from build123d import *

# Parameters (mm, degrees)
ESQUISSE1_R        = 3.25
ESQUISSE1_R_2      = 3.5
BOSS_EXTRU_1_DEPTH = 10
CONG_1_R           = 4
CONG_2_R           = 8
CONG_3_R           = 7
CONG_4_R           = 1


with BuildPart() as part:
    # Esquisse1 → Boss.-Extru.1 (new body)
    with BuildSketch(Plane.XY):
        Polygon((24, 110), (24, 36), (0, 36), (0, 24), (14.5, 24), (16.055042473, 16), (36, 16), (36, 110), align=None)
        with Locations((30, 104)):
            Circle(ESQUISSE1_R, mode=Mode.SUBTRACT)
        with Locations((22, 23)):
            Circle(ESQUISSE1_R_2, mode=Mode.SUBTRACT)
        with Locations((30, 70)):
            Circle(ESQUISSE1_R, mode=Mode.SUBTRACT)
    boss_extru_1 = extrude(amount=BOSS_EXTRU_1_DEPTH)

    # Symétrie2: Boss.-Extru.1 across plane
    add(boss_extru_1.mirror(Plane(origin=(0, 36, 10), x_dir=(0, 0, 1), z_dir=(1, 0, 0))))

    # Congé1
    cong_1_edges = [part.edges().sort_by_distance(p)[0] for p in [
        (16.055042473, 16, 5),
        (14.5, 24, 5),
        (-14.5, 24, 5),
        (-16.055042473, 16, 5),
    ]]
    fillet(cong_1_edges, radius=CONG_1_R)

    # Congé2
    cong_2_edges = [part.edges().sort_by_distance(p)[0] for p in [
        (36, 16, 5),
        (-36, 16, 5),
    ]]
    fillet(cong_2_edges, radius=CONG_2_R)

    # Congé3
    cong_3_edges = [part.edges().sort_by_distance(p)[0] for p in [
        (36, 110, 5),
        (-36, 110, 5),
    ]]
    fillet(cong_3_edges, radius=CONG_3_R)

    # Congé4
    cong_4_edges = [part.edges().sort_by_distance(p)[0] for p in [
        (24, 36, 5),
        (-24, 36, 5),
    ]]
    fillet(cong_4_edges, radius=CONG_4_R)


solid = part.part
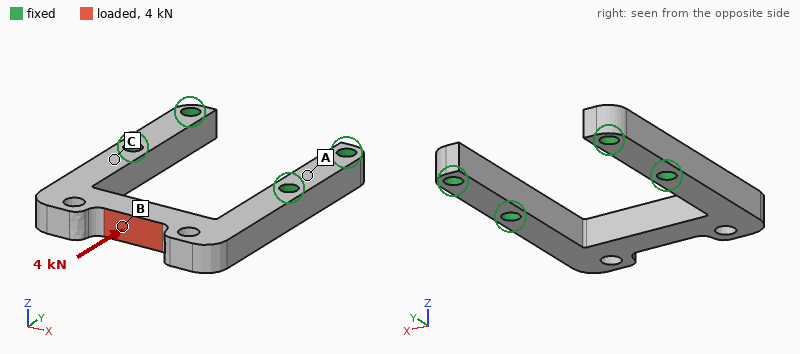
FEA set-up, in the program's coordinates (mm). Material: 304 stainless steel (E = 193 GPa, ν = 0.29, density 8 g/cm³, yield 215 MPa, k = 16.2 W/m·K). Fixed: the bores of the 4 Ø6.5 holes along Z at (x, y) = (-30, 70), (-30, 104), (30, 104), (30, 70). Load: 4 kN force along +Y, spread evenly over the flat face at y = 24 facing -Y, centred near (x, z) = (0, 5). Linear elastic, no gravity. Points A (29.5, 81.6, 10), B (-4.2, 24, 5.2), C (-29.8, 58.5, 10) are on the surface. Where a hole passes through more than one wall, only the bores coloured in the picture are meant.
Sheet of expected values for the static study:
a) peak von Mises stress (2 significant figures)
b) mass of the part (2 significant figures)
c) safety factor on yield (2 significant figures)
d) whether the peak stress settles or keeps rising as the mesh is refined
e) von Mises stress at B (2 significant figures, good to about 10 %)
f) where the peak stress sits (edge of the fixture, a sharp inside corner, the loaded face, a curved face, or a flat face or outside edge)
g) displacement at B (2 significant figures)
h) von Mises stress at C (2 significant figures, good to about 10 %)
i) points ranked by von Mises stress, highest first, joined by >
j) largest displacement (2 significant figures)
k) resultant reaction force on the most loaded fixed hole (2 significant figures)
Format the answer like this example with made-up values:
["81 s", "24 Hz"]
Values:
["250 MPa", "220 g", "0.86", "settles", "100 MPa", "a curved face", "28 µm", "27 MPa", "B > C > A", "30 µm", "2.2 kN"]
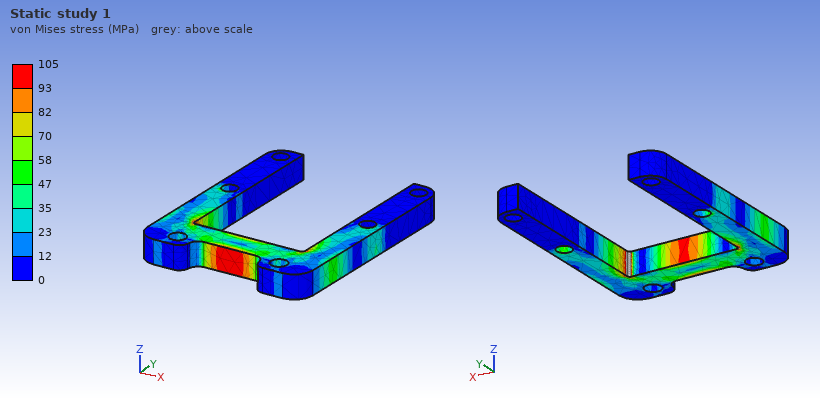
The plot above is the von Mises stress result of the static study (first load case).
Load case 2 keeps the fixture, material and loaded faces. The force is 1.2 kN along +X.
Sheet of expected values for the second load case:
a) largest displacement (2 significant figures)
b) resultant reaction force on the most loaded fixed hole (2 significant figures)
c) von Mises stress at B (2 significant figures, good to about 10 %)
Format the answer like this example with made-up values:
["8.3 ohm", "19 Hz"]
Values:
["19 µm", "800 N", "9.4 MPa"]
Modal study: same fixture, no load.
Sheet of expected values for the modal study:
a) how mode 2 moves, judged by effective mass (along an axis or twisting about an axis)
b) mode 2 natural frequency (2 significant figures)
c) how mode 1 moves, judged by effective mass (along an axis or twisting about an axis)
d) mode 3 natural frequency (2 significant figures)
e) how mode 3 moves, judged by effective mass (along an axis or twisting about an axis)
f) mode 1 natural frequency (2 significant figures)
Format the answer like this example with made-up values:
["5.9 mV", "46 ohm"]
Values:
["twisting about Y", "3800 Hz", "along Z", "4000 Hz", "along X", "2100 Hz"]
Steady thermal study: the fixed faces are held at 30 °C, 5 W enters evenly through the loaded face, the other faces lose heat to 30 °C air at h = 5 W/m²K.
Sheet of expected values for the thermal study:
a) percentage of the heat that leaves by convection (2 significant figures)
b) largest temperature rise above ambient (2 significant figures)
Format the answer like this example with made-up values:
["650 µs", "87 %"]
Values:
["22 %", "65 K"]
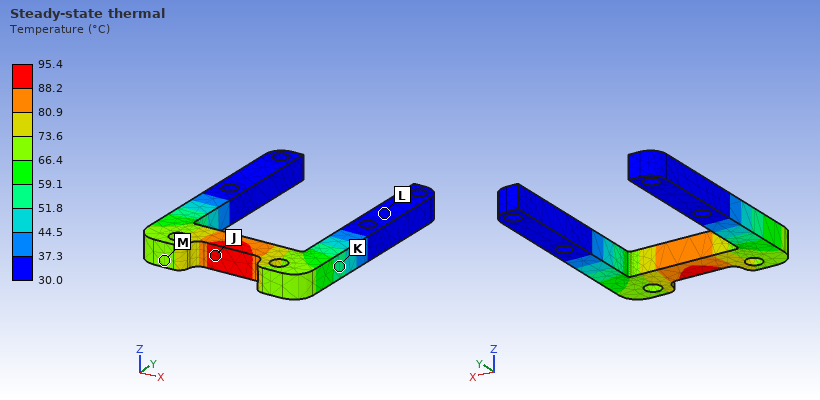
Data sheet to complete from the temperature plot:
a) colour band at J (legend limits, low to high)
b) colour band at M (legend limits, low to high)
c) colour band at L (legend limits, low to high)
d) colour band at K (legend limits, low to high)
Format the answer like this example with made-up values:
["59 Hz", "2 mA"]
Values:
["88.2 to 95.4 °C", "66.4 to 73.6 °C", "30.0 to 37.3 °C", "51.8 to 59.1 °C"]
